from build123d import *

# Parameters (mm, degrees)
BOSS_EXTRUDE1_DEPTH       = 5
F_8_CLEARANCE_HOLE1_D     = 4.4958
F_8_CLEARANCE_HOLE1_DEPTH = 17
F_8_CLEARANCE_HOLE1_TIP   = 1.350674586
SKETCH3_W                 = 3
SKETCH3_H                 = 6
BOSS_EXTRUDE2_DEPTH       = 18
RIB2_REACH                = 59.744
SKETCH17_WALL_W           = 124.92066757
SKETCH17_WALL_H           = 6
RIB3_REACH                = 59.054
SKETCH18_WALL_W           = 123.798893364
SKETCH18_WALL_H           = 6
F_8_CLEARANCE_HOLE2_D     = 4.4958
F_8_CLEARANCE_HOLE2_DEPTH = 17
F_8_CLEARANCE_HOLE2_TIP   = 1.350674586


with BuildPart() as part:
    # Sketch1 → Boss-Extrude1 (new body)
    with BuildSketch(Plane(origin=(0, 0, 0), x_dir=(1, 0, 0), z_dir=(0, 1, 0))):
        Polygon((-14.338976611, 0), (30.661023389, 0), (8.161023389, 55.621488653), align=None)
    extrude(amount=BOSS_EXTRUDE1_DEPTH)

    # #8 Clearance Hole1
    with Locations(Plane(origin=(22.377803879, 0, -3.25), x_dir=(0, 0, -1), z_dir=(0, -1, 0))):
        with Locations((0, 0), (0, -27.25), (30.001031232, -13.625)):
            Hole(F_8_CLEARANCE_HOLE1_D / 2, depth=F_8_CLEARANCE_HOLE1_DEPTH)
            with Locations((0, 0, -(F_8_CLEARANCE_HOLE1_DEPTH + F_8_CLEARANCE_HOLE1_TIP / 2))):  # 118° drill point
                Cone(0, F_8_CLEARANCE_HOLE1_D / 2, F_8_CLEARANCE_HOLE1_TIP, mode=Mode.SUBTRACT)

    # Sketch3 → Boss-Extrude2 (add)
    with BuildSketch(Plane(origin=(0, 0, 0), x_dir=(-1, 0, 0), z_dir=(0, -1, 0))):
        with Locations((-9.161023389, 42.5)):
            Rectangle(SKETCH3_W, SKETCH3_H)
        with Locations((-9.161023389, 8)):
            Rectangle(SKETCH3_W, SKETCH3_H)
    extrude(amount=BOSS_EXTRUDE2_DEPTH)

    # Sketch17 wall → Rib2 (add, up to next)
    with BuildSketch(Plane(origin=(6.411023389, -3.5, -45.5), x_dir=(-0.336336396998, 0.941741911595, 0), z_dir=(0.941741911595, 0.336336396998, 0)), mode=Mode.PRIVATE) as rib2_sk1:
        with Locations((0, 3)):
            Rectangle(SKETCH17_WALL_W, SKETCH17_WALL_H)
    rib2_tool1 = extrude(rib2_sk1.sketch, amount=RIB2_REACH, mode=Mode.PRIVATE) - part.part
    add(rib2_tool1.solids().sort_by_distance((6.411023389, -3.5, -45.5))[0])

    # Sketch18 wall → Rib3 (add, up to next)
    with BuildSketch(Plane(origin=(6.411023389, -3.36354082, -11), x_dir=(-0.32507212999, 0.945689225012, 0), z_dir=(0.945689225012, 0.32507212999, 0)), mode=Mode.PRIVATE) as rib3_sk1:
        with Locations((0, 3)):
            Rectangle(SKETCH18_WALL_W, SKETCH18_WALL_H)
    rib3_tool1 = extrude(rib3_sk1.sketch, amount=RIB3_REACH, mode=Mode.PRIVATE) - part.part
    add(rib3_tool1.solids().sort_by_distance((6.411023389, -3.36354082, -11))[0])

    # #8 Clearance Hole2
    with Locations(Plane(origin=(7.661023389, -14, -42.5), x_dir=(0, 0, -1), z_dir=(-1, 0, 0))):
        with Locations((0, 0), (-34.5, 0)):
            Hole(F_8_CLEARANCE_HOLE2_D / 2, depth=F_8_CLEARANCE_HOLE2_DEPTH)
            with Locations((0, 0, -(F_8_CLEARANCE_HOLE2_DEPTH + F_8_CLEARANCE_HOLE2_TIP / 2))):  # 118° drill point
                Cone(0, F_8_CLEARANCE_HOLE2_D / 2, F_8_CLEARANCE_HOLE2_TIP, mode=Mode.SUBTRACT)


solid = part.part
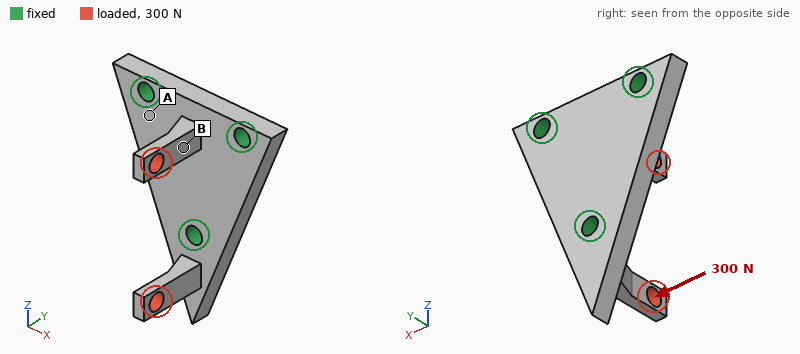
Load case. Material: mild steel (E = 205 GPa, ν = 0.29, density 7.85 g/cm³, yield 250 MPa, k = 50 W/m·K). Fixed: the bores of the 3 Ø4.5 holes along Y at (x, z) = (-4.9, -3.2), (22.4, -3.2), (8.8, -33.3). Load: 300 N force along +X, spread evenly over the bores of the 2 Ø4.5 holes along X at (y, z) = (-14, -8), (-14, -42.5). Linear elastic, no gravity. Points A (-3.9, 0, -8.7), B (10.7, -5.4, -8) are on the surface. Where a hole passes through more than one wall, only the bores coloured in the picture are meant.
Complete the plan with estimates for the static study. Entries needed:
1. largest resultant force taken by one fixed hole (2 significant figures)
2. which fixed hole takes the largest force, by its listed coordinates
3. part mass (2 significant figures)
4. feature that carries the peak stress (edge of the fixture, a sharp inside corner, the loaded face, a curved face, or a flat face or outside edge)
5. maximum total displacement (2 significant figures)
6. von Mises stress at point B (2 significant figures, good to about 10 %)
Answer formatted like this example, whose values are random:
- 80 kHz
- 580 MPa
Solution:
- 180 N
- (8.8, -33.3)
- 52 g
- a flat face or outside edge
- 52 µm
- 110 MPa
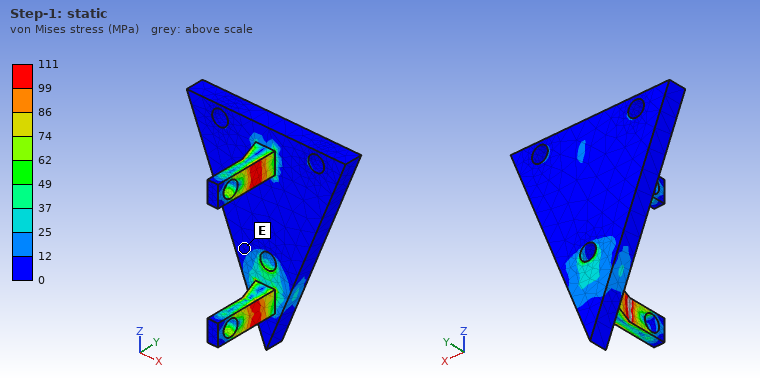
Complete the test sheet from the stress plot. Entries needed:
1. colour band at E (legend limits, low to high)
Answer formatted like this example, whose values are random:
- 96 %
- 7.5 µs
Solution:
- 0 to 12 MPa
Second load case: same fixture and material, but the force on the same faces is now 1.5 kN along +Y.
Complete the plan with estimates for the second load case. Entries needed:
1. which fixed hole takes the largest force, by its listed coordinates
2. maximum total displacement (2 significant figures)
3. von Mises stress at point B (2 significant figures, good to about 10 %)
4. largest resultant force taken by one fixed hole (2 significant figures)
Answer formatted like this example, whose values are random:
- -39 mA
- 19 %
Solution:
- (8.8, -33.3)
- 25 µm
- 49 MPa
- 880 N
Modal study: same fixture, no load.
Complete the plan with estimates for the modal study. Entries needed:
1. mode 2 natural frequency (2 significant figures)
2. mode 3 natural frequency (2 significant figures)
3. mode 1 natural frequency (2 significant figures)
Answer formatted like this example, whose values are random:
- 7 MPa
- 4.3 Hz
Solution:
- 11 kHz
- 12 kHz
- 10 kHz
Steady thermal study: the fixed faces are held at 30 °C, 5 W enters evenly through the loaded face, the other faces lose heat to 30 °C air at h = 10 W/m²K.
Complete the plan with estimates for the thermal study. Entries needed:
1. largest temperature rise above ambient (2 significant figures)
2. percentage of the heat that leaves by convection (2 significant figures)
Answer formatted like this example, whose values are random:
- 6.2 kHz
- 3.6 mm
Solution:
- 55 K
- 4.7 %
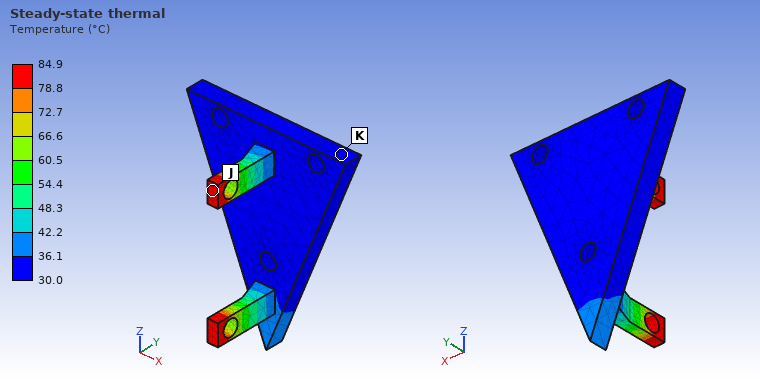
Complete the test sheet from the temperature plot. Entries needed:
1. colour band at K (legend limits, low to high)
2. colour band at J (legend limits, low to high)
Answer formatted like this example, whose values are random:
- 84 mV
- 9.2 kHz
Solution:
- 30.0 to 36.1 °C
- 78.8 to 84.9 °C
